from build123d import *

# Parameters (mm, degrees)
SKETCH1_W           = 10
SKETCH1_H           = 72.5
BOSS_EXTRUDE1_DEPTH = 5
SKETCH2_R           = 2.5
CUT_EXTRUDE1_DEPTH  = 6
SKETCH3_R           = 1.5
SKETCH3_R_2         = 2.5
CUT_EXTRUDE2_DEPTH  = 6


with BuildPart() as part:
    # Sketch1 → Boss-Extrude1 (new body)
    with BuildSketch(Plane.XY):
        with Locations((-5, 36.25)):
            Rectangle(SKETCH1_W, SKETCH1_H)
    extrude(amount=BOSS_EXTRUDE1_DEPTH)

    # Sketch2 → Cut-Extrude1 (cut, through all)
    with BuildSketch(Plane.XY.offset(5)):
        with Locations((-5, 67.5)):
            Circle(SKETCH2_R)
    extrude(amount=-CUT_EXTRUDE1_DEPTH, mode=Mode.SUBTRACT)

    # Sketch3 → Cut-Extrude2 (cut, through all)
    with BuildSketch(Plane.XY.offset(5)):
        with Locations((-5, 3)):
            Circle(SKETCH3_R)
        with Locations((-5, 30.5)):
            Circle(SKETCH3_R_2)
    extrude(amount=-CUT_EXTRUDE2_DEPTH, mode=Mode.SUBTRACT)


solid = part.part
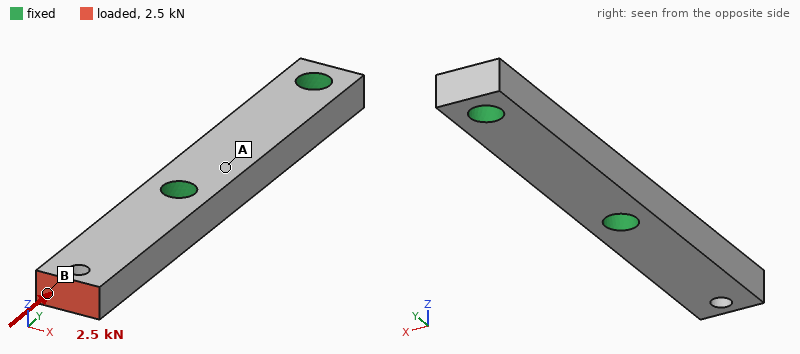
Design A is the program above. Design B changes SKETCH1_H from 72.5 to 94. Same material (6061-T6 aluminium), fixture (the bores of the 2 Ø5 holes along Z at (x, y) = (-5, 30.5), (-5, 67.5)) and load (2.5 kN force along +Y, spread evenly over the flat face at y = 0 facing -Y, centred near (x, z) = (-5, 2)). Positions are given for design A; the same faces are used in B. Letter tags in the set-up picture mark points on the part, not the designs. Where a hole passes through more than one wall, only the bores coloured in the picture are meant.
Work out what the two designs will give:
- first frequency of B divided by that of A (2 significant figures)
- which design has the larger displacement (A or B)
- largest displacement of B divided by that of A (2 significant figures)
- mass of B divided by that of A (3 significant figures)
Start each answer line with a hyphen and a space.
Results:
- 0.52
- B
- 1.2
- 1.32
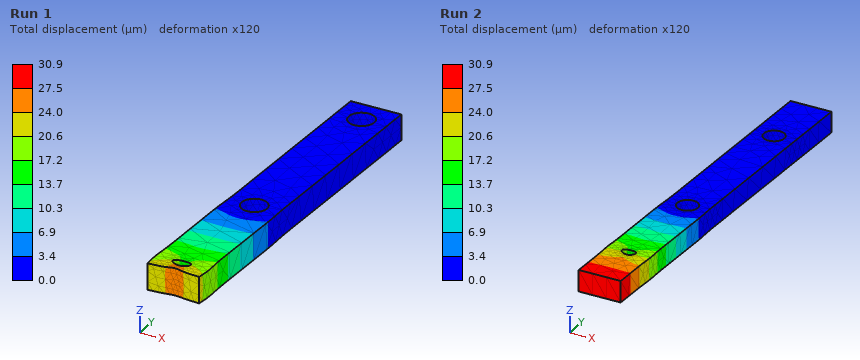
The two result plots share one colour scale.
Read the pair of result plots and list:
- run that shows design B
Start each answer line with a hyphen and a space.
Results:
- Run 2
